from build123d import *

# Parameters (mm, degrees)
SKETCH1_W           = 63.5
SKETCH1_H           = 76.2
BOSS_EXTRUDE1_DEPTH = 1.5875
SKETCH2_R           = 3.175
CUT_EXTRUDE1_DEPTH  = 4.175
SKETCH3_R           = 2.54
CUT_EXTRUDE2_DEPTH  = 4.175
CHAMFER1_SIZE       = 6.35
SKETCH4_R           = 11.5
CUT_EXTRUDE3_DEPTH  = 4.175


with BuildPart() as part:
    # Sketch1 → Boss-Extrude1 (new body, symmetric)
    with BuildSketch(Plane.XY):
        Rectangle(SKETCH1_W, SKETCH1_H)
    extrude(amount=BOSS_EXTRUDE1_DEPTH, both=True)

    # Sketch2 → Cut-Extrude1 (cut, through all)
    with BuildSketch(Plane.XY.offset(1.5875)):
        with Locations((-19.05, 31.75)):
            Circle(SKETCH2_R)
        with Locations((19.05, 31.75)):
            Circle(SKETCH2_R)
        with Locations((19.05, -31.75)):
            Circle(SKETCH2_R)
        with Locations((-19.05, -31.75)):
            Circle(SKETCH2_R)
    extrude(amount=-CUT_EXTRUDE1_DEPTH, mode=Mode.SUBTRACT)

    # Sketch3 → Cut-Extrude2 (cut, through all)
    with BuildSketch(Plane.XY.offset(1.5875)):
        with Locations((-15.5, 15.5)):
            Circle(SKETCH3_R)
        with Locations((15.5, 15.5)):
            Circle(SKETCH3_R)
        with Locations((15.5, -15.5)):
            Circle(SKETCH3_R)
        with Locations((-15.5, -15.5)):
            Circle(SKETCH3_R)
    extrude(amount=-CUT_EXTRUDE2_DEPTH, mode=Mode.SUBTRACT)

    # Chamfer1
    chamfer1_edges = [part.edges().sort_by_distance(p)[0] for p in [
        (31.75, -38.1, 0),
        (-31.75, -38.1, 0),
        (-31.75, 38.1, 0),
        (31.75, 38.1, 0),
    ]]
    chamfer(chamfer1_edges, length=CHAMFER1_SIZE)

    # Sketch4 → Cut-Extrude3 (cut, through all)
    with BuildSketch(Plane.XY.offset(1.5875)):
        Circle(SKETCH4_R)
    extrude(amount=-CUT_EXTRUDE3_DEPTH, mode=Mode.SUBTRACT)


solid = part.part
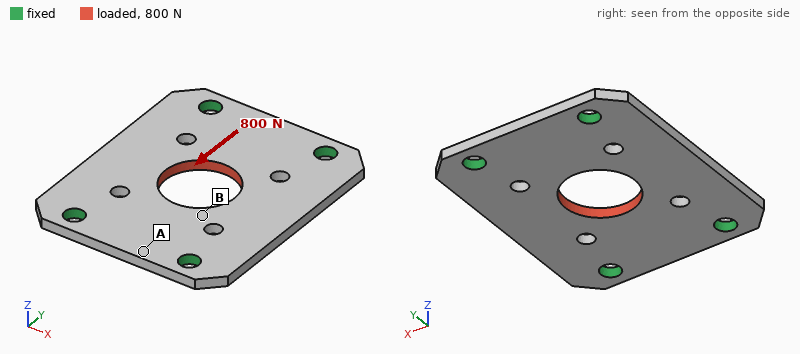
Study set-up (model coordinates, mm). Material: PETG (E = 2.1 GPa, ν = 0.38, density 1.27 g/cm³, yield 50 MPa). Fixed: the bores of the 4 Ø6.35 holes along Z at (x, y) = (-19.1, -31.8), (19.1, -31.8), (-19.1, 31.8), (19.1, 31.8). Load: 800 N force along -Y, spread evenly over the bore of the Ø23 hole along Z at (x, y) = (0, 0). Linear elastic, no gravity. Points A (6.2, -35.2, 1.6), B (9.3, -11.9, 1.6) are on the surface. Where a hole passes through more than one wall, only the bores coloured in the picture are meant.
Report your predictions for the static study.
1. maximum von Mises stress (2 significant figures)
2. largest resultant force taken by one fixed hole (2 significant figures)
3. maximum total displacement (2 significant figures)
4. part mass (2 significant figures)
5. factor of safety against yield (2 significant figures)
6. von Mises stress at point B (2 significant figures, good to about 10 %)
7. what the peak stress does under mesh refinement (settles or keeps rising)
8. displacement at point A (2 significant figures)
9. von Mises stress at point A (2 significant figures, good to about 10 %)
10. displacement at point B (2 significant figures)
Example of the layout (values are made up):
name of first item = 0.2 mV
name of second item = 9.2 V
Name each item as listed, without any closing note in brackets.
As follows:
maximum von Mises stress = 10 MPa
largest resultant force taken by one fixed hole = 210 N
maximum total displacement = 56 µm
part mass = 17 g
factor of safety against yield = 4.9
von Mises stress at point B = 4.4 MPa
what the peak stress does under mesh refinement = settles
displacement at point A = 28 µm
von Mises stress at point A = 1.2 MPa
displacement at point B = 44 µm
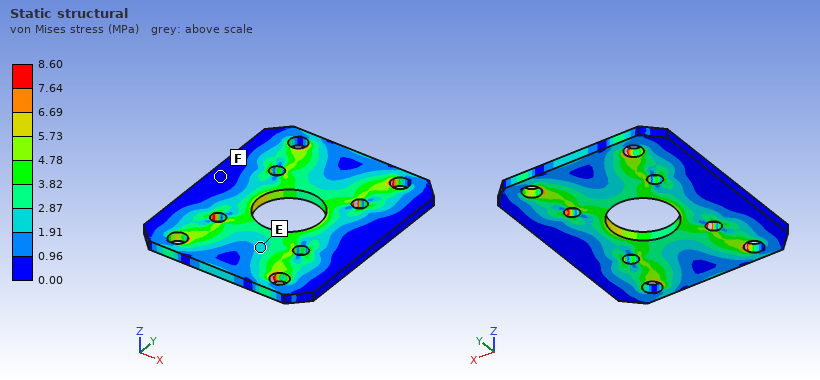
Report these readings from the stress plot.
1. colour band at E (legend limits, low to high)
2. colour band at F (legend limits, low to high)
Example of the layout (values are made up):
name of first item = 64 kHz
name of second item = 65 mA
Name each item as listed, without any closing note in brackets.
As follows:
colour band at E = 1.91 to 2.87 MPa
colour band at F = 0.00 to 0.96 MPa
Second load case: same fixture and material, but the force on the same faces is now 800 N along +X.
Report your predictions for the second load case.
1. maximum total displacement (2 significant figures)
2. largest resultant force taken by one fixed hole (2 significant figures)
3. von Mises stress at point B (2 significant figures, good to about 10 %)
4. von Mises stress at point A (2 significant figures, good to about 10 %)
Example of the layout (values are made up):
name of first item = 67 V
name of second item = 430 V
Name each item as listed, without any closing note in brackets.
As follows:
maximum total displacement = 0.11 mm
largest resultant force taken by one fixed hole = 220 N
von Mises stress at point B = 3.8 MPa
von Mises stress at point A = 1.1 MPa
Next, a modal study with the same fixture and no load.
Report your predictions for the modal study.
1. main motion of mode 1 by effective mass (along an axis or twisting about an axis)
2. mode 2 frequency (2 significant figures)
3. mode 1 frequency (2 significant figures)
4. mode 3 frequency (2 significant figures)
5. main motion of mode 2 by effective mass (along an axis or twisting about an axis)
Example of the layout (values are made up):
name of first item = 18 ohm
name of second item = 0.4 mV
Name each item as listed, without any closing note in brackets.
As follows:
main motion of mode 1 by effective mass = along Z
mode 2 frequency = 1200 Hz
mode 1 frequency = 1100 Hz
mode 3 frequency = 1800 Hz
main motion of mode 2 by effective mass = twisting about Y
